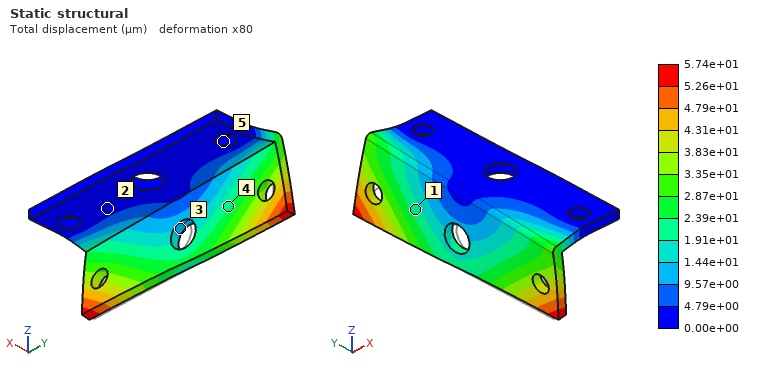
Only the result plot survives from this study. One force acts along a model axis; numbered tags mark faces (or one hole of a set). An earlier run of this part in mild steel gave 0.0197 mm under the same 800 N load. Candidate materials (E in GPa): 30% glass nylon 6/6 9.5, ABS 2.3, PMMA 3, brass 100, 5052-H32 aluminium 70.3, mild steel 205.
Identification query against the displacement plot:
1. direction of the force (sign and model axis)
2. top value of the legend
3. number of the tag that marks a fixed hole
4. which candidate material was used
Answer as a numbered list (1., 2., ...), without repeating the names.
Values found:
1. +Y
2. 5.74e+01 µm
3. 5
4. 5052-H32 aluminium
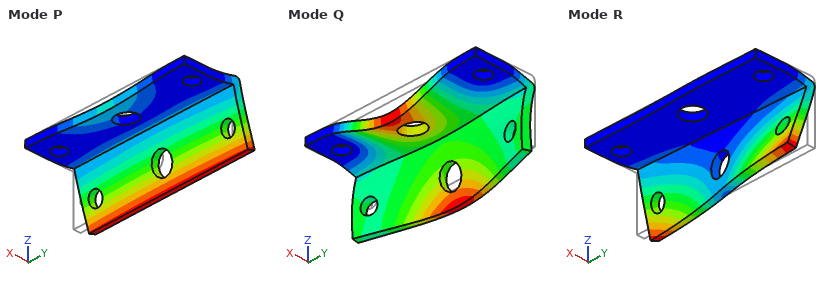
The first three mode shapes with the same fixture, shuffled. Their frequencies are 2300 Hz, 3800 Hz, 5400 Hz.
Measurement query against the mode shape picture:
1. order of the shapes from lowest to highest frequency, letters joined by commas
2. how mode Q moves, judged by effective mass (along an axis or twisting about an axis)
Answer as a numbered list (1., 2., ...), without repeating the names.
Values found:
1. P, R, Q
2. along Z
